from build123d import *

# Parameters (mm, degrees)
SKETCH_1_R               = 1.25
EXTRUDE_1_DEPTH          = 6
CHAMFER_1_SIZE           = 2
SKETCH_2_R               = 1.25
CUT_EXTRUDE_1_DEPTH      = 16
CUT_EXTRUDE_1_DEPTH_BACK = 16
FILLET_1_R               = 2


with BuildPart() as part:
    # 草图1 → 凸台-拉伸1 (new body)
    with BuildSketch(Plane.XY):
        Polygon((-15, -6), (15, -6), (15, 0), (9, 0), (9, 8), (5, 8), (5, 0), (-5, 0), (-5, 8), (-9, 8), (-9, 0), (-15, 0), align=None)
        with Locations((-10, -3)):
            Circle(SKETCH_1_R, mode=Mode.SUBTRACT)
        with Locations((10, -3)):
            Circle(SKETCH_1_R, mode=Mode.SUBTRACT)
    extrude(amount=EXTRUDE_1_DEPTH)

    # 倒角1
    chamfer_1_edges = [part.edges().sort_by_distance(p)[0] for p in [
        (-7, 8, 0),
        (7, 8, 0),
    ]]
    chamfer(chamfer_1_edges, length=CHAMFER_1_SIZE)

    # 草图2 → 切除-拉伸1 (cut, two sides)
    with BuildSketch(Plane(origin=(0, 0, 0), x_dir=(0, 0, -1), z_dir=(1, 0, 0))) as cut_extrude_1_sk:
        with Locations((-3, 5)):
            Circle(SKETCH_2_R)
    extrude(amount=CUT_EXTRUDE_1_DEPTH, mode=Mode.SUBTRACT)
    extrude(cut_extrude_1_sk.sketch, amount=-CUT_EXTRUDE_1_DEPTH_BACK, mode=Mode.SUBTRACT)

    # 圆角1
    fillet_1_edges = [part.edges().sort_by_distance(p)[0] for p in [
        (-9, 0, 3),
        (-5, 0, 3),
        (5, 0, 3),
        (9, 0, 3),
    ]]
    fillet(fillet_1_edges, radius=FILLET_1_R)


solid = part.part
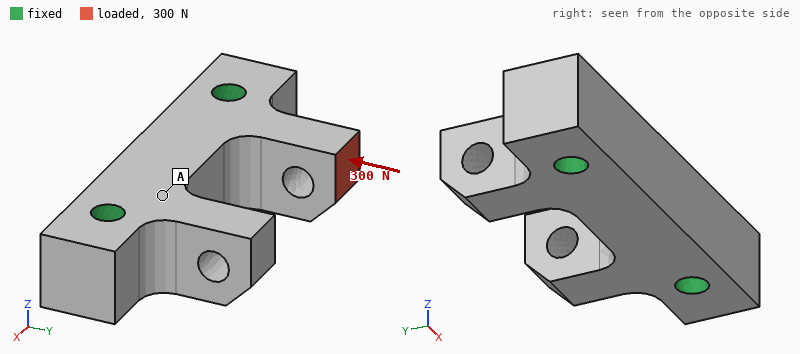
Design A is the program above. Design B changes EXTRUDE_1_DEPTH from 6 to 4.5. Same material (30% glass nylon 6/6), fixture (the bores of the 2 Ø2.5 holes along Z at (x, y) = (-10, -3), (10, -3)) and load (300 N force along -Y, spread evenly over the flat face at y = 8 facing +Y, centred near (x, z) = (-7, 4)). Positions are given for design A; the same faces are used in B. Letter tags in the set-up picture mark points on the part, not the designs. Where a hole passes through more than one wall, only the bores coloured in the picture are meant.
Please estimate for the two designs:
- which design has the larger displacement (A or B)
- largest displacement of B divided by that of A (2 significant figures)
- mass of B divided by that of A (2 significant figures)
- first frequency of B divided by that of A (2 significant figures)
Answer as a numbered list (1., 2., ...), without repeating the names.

1. B
2. 2.8
3. 0.74
4. 0.97
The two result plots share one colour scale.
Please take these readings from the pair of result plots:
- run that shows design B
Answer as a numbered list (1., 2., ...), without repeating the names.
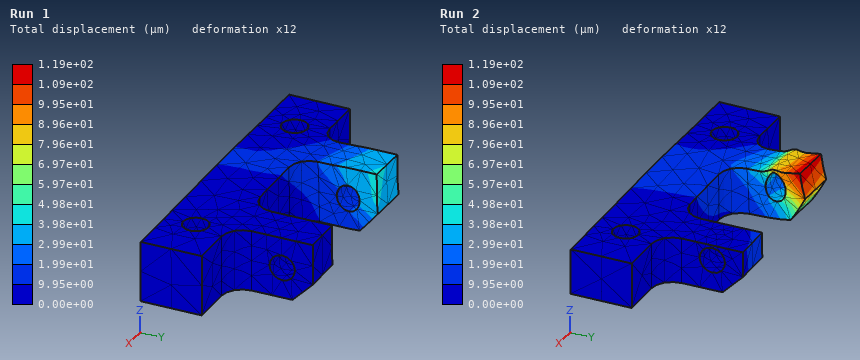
1. Run 2
